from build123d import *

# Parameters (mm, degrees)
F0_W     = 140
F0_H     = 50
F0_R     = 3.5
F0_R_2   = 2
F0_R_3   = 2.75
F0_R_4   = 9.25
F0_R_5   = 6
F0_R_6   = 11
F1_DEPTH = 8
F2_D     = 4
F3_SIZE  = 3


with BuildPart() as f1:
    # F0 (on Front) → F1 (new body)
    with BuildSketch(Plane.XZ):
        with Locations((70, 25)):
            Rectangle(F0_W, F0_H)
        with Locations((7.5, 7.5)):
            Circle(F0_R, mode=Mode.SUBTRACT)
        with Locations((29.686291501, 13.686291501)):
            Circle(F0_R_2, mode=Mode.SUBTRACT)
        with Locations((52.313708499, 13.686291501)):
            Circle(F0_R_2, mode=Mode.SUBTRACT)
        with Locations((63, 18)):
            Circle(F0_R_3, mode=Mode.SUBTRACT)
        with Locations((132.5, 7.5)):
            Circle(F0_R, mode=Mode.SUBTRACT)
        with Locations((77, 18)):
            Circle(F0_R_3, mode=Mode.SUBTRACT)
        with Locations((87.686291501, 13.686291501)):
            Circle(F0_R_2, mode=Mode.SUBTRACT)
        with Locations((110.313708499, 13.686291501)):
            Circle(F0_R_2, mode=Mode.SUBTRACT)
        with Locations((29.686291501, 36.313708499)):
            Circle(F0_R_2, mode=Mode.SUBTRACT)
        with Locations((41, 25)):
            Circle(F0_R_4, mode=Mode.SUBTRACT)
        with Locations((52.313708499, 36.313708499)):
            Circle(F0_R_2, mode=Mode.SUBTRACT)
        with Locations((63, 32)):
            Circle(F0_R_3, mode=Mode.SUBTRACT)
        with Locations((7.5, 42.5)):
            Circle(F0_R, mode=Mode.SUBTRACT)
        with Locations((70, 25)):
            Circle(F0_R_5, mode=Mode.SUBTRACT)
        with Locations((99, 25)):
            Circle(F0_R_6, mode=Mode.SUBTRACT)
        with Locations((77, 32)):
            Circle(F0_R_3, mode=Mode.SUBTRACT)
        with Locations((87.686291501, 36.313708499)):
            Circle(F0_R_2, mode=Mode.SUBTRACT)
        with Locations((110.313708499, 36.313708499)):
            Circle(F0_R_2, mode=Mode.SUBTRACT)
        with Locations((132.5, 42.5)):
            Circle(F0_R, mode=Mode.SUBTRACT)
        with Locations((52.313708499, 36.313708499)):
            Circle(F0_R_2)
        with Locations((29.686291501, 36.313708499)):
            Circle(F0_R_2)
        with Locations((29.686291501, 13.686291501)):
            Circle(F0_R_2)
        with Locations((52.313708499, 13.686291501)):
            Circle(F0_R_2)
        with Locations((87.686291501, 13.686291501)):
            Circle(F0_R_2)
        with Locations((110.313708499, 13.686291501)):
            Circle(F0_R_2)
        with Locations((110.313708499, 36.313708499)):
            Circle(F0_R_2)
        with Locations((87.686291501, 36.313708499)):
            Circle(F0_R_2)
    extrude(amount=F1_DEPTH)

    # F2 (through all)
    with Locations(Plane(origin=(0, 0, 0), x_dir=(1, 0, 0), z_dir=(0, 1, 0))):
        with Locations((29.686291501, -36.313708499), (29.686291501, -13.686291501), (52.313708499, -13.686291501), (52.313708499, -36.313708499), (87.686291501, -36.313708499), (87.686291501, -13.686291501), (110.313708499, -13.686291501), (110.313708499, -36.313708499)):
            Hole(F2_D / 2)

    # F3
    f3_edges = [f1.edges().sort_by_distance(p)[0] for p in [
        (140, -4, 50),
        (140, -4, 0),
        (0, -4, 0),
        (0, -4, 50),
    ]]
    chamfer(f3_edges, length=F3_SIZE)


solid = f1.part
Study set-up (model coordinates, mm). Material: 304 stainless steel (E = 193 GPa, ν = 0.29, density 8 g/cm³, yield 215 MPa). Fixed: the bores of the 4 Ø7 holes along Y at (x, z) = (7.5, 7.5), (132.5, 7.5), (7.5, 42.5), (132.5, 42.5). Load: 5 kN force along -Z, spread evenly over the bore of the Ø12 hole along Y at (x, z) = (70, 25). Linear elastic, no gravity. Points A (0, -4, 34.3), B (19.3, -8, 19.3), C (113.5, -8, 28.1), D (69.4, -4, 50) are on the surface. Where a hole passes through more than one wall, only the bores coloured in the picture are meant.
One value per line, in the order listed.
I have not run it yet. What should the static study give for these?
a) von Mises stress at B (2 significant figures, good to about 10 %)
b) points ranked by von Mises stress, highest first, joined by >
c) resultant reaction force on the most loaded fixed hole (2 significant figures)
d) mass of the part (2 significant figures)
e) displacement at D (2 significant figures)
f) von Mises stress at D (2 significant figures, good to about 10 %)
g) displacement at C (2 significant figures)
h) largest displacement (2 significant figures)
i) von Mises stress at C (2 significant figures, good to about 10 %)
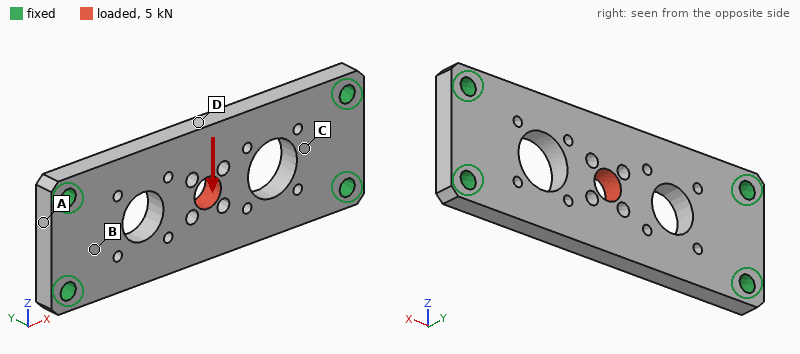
20 MPa
D > C > B > A
2.6 kN
380 g
15 µm
34 MPa
2.5 µm
16 µm
27 MPa
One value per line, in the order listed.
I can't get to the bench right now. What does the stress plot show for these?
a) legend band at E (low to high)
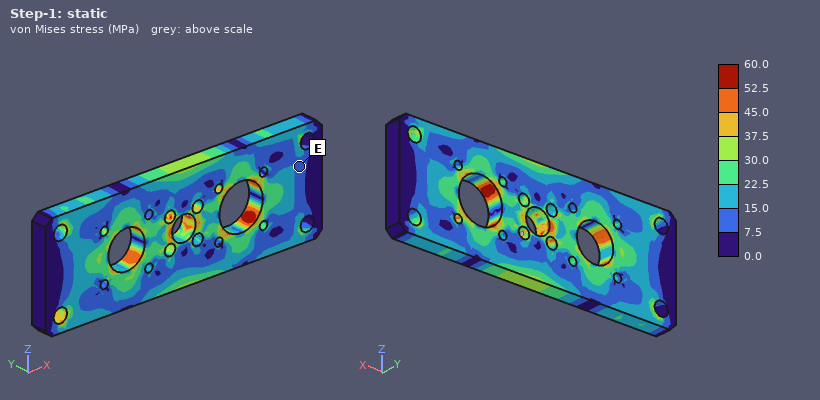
7.5 to 15.0 MPa
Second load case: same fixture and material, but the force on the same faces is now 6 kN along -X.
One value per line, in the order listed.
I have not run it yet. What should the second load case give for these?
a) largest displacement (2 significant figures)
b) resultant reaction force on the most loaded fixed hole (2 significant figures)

6.7 µm
1.6 kN
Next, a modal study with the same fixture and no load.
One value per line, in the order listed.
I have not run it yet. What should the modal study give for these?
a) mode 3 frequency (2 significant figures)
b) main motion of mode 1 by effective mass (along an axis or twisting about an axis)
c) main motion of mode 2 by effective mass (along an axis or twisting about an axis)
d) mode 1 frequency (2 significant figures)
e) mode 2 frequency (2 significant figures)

6800 Hz
along Y
twisting about X
2600 Hz
4300 Hz
